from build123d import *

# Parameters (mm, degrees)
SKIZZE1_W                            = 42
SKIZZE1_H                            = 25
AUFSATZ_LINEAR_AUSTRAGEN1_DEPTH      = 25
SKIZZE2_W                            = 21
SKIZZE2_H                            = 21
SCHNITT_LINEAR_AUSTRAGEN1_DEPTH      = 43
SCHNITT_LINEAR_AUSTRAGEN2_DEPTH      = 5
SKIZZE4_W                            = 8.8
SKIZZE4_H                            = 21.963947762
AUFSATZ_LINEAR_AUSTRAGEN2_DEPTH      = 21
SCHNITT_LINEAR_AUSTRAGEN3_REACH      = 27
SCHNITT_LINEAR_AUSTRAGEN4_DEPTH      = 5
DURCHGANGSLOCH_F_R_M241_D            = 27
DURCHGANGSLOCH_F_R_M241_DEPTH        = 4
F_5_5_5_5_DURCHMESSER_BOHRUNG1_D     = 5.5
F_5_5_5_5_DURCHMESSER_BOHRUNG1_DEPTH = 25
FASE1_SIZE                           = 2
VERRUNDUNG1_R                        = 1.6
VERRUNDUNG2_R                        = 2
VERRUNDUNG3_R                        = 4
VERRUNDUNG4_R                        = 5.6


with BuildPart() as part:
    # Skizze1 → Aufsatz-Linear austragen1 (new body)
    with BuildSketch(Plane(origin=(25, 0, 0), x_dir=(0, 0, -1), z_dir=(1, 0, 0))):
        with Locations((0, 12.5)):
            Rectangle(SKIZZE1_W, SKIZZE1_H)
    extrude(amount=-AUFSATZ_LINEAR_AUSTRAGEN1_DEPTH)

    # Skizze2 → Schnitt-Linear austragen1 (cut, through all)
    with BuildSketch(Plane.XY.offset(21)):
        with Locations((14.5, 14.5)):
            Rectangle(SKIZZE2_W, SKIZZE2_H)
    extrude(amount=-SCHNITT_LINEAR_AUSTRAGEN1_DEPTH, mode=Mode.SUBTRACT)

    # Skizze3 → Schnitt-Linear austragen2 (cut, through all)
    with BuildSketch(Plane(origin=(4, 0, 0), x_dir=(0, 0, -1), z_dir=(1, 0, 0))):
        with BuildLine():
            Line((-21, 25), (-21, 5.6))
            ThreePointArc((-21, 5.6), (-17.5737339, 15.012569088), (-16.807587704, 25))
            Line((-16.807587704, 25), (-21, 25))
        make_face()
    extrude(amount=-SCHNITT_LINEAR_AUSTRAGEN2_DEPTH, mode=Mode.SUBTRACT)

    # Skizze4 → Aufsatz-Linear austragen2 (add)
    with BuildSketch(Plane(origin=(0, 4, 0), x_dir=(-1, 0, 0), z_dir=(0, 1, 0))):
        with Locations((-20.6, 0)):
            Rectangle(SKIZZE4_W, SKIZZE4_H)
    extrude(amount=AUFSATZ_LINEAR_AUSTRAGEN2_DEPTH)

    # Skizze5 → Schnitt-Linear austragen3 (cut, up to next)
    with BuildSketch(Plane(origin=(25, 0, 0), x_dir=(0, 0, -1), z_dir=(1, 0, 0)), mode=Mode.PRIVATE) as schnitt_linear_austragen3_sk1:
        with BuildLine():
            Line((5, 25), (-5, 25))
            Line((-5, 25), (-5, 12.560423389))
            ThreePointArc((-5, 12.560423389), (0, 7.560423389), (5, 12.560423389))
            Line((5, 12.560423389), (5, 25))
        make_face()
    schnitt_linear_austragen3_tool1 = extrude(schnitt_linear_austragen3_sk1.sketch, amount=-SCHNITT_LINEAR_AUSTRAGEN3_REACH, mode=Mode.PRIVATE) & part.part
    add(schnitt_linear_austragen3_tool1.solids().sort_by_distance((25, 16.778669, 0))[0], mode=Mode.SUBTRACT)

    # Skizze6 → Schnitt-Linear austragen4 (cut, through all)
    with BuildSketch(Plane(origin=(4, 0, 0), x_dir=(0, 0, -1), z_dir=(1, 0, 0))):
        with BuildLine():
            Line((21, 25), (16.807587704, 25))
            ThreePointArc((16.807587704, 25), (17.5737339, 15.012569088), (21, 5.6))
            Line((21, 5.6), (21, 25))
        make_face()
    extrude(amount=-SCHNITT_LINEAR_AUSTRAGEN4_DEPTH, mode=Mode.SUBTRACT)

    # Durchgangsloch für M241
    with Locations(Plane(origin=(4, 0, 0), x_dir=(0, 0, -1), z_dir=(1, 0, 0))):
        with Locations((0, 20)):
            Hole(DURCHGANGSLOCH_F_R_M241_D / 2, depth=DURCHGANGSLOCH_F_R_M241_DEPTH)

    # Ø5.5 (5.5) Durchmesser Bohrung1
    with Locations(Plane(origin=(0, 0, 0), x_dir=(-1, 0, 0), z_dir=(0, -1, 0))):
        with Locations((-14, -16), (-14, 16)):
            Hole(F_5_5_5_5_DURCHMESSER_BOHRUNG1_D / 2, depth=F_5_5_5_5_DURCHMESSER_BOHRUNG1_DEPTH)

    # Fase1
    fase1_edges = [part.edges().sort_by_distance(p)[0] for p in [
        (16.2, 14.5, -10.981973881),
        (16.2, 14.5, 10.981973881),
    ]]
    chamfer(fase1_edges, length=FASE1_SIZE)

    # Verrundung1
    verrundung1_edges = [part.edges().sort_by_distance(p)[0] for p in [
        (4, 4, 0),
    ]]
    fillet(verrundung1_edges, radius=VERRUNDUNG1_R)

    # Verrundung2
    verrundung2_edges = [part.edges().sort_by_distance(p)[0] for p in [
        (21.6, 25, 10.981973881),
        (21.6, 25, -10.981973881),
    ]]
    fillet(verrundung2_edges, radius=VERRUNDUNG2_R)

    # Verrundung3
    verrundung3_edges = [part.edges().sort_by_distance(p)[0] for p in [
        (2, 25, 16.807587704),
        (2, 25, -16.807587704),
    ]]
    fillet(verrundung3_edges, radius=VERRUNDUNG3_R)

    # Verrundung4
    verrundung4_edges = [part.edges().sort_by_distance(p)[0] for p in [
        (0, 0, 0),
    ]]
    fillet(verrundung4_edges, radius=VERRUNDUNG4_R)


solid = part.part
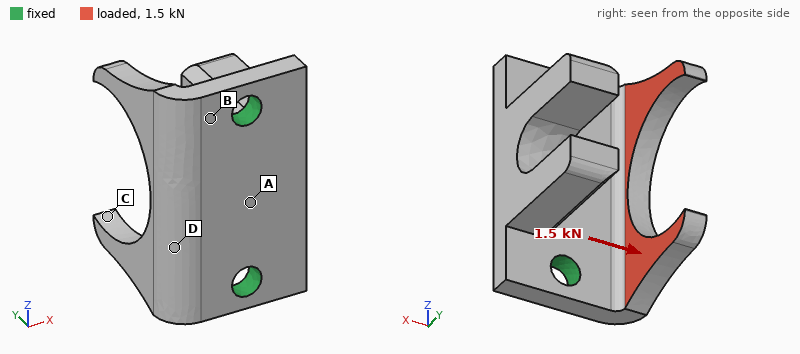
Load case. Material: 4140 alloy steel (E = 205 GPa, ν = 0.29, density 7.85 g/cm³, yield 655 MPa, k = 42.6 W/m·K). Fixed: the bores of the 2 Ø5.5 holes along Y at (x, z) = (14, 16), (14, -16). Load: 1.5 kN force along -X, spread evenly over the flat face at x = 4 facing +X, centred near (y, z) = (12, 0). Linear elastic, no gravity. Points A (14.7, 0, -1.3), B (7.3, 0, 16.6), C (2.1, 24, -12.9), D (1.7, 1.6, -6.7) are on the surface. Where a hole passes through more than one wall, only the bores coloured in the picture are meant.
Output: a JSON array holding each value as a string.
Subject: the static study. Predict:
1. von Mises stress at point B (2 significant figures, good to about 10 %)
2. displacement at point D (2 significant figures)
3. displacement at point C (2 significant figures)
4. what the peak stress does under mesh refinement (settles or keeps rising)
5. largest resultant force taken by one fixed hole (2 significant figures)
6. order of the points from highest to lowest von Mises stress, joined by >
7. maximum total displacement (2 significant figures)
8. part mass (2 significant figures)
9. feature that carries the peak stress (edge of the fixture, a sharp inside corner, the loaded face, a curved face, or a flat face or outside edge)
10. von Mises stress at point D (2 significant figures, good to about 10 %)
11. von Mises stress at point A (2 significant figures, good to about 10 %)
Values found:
["130 MPa", "0.023 mm", "0.13 mm", "keeps rising", "750 N", "B > D > A > C", "0.14 mm", "60 g", "edge of the fixture", "69 MPa", "44 MPa"]
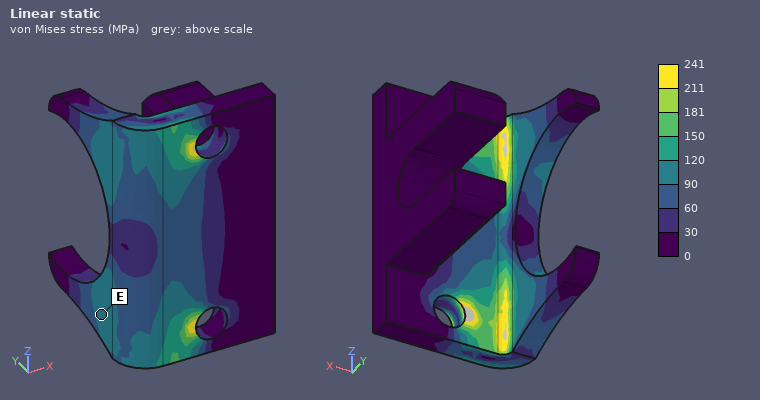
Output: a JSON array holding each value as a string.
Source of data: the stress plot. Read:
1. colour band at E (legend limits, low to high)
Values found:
["90 to 120 MPa"]
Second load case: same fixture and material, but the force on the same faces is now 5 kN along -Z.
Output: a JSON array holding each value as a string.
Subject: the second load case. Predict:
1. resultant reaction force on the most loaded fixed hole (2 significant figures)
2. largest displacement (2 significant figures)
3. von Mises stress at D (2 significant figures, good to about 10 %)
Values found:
["3.2 kN", "0.13 mm", "100 MPa"]
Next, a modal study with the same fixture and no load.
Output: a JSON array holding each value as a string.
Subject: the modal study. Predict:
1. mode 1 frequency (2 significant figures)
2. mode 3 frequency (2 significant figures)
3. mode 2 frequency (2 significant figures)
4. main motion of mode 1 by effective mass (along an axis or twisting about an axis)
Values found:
["6000 Hz", "8000 Hz", "7300 Hz", "along X"]
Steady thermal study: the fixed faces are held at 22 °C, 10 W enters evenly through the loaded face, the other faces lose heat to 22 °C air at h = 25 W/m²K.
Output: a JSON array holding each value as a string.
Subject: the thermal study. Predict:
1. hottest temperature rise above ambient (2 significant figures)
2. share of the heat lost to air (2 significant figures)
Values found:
["44 K", "10 %"]
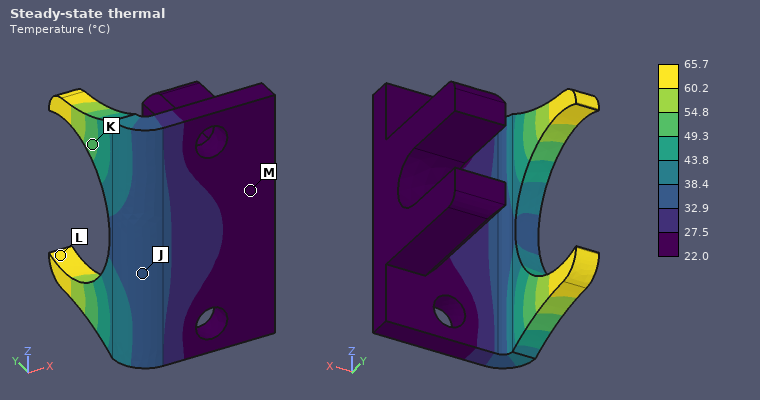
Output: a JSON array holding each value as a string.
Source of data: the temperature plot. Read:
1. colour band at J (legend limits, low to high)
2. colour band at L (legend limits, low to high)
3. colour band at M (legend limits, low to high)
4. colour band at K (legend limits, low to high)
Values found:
["32.9 to 38.4 °C", "60.2 to 65.7 °C", "22.0 to 27.5 °C", "49.3 to 54.8 °C"]
